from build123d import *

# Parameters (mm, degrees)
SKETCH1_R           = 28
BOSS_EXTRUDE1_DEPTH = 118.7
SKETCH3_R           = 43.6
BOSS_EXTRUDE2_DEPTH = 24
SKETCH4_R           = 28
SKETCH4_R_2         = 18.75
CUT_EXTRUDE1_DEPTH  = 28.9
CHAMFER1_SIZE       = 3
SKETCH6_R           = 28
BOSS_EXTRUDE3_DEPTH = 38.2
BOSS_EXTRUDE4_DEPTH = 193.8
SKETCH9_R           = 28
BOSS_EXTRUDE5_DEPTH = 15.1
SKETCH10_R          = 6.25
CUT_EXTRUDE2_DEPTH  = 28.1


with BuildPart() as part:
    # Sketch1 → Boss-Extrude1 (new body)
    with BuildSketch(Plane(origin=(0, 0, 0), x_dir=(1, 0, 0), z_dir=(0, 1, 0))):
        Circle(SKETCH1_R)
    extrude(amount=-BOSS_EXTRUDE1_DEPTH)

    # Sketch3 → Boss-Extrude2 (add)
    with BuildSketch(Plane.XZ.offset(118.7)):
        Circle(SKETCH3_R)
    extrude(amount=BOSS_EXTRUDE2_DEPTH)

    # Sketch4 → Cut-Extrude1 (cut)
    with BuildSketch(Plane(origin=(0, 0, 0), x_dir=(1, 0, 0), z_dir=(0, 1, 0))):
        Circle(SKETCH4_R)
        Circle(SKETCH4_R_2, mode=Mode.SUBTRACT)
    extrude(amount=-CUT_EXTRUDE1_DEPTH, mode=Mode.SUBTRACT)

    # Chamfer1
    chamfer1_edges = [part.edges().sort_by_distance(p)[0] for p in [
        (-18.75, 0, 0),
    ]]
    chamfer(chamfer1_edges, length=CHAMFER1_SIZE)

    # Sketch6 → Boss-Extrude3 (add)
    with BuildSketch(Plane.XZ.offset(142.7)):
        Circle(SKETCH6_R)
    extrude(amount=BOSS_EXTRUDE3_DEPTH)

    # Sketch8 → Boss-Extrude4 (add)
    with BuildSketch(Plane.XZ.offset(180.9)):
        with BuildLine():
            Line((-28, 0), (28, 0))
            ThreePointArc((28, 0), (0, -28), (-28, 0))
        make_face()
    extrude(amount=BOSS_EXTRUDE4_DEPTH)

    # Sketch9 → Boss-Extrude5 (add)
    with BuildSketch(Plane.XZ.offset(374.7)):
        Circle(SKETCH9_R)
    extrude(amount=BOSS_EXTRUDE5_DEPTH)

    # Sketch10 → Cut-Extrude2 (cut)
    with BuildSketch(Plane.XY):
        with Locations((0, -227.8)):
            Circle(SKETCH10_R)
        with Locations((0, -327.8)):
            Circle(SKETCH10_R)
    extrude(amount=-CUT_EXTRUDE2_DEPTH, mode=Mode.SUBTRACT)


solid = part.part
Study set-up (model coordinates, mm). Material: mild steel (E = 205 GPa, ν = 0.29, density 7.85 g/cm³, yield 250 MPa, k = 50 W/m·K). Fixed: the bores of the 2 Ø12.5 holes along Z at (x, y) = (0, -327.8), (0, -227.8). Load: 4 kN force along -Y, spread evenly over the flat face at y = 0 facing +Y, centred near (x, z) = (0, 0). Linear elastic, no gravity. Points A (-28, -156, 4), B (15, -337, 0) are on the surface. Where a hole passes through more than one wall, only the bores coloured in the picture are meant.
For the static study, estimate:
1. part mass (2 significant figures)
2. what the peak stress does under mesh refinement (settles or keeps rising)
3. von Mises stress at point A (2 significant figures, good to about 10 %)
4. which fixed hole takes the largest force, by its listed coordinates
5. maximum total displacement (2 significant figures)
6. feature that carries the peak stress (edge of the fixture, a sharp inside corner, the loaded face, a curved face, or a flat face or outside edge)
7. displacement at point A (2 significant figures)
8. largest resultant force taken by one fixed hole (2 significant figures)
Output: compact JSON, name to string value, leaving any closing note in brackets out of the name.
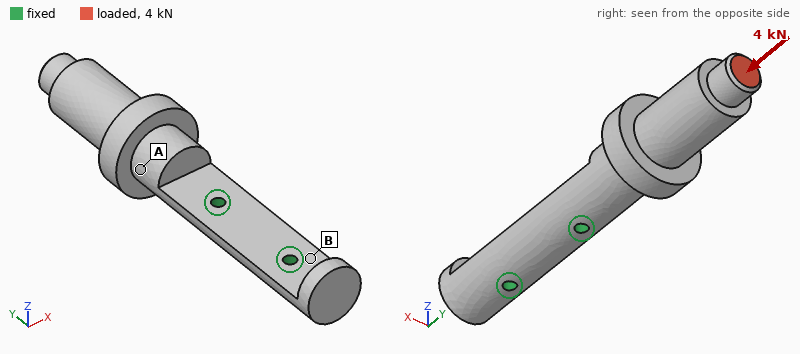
{"part mass": "6.0 kg", "what the peak stress does under mesh refinement": "keeps rising", "von Mises stress at point A": "2.7 MPa", "which fixed hole takes the largest force, by its listed coordinates": "(0, -227.8)", "maximum total displacement": "41 µm", "feature that carries the peak stress": "edge of the fixture", "displacement at point A": "9.7 µm", "largest resultant force taken by one fixed hole": "3.6 kN"}
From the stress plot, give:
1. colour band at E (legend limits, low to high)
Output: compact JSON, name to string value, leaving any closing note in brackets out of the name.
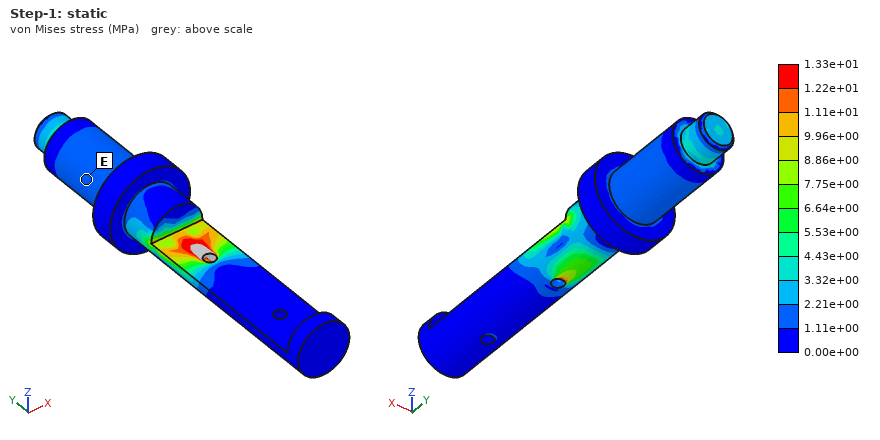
{"colour band at E": "1.11e+00 to 2.21e+00 MPa"}
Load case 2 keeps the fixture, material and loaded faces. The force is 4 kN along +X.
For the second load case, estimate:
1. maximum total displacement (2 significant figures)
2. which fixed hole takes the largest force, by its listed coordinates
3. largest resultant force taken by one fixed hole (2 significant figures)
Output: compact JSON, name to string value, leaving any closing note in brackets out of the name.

{"maximum total displacement": "0.34 mm", "which fixed hole takes the largest force, by its listed coordinates": "(0, -227.8)", "largest resultant force taken by one fixed hole": "9.4 kN"}
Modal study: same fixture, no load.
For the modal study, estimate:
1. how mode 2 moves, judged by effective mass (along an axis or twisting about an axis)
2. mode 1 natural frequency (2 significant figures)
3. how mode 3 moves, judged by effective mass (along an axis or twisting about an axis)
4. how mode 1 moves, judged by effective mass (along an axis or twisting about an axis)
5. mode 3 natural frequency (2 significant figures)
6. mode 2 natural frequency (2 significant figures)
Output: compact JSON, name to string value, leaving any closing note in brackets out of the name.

{"how mode 2 moves, judged by effective mass": "along X", "mode 1 natural frequency": "360 Hz", "how mode 3 moves, judged by effective mass": "twisting about Y", "how mode 1 moves, judged by effective mass": "along Z", "mode 3 natural frequency": "1700 Hz", "mode 2 natural frequency": "520 Hz"}
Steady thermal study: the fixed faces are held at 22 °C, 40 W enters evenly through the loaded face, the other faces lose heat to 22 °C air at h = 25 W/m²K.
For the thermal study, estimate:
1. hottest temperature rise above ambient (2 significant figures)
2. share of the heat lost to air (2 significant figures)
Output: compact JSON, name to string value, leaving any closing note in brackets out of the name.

{"hottest temperature rise above ambient": "64 K", "share of the heat lost to air": "67 %"}
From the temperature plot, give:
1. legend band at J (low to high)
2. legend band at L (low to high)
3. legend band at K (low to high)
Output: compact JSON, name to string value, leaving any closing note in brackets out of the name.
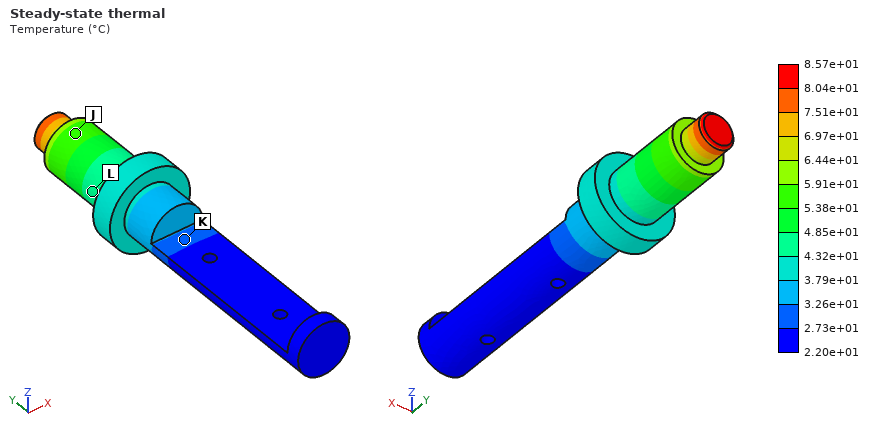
{"legend band at J": "5.38e+01 to 5.91e+01 °C", "legend band at L": "4.32e+01 to 4.85e+01 °C", "legend band at K": "2.73e+01 to 3.26e+01 °C"}
